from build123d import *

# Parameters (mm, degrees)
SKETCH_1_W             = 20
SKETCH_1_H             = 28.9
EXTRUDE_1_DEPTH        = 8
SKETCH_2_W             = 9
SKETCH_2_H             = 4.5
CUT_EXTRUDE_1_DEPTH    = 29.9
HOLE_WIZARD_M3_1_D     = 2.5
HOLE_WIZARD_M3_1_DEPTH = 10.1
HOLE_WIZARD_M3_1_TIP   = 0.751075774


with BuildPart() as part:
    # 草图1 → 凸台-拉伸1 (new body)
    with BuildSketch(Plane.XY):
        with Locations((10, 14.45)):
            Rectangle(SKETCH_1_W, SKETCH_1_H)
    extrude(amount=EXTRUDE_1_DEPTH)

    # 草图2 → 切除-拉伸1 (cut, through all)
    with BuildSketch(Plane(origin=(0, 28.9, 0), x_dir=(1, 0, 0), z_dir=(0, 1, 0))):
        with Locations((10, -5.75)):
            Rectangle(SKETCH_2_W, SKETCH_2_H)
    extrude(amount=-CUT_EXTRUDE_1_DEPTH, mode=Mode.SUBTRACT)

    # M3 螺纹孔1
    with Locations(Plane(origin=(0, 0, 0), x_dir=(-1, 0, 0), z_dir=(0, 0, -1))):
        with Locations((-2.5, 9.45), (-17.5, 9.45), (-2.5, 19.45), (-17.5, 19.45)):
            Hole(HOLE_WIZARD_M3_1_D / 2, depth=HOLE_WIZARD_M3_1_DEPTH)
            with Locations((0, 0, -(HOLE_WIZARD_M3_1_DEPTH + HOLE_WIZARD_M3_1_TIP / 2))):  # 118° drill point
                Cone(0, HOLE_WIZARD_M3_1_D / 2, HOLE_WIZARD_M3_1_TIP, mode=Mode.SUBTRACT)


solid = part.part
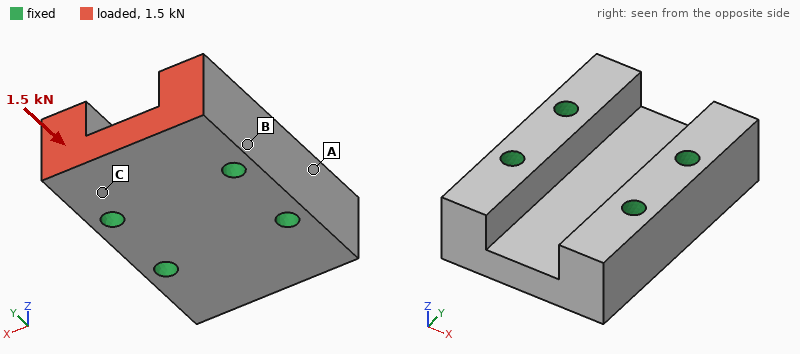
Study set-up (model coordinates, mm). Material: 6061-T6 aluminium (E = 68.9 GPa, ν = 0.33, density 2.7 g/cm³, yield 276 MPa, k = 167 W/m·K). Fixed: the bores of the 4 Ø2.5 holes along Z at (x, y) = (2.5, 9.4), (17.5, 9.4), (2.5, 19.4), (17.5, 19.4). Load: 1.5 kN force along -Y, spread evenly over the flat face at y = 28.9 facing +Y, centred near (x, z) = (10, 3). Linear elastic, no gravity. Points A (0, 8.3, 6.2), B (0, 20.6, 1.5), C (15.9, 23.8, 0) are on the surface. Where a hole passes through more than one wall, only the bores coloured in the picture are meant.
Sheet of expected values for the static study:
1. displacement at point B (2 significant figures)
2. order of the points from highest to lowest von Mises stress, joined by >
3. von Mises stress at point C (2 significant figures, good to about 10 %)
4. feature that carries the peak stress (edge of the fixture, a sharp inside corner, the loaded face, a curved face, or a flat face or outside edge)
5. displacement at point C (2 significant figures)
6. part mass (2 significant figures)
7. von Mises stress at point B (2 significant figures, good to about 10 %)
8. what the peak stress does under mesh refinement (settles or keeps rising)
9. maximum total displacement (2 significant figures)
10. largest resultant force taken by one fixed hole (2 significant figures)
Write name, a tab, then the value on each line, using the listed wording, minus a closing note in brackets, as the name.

displacement at point B	0.41 µm
order of the points from highest to lowest von Mises stress, joined by >	C > B > A
von Mises stress at point C	15 MPa
feature that carries the peak stress	edge of the fixture
displacement at point C	1.1 µm
part mass	8.9 g
von Mises stress at point B	8.8 MPa
what the peak stress does under mesh refinement	keeps rising
maximum total displacement	2.3 µm
largest resultant force taken by one fixed hole	670 N
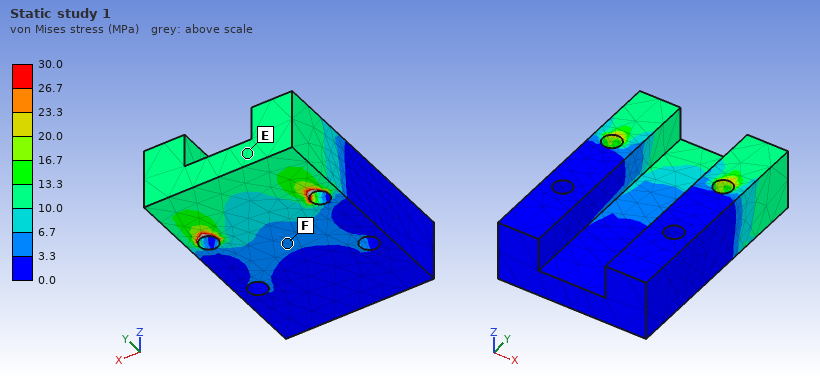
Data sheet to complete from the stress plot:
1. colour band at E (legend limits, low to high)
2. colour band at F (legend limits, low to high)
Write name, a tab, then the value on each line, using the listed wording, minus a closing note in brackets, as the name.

colour band at E	10.0 to 13.3 MPa
colour band at F	3.3 to 6.7 MPa
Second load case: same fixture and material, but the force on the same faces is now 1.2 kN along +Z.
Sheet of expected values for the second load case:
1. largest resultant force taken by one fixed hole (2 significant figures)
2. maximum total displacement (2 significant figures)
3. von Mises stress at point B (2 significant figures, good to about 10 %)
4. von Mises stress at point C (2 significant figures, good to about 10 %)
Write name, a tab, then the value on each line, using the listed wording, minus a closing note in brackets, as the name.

largest resultant force taken by one fixed hole	650 N
maximum total displacement	18 µm
von Mises stress at point B	21 MPa
von Mises stress at point C	43 MPa
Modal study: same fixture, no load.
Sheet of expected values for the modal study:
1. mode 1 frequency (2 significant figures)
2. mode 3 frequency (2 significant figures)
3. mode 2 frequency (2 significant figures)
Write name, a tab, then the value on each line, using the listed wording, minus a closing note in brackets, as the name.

mode 1 frequency	47 kHz
mode 3 frequency	55 kHz
mode 2 frequency	48 kHz
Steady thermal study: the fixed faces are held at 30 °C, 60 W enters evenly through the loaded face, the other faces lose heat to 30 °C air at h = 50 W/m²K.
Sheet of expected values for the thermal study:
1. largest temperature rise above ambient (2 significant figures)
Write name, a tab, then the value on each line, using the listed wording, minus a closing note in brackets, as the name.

largest temperature rise above ambient	29 K
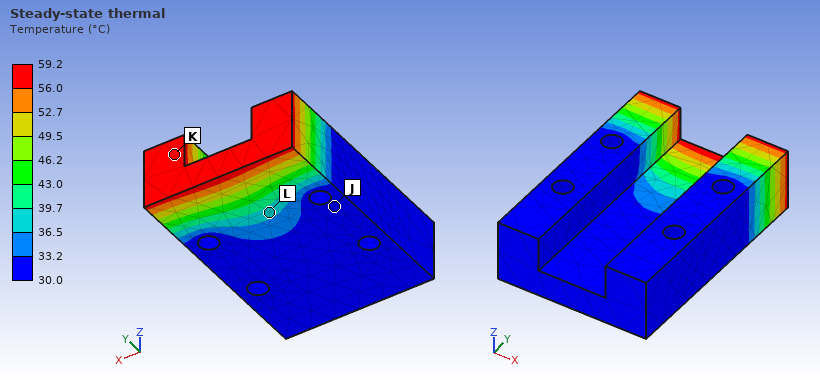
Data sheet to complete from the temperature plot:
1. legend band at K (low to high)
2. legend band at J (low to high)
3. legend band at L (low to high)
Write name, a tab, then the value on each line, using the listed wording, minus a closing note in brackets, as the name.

legend band at K	56.0 to 59.2 °C
legend band at J	30.0 to 33.2 °C
legend band at L	36.5 to 39.7 °C
